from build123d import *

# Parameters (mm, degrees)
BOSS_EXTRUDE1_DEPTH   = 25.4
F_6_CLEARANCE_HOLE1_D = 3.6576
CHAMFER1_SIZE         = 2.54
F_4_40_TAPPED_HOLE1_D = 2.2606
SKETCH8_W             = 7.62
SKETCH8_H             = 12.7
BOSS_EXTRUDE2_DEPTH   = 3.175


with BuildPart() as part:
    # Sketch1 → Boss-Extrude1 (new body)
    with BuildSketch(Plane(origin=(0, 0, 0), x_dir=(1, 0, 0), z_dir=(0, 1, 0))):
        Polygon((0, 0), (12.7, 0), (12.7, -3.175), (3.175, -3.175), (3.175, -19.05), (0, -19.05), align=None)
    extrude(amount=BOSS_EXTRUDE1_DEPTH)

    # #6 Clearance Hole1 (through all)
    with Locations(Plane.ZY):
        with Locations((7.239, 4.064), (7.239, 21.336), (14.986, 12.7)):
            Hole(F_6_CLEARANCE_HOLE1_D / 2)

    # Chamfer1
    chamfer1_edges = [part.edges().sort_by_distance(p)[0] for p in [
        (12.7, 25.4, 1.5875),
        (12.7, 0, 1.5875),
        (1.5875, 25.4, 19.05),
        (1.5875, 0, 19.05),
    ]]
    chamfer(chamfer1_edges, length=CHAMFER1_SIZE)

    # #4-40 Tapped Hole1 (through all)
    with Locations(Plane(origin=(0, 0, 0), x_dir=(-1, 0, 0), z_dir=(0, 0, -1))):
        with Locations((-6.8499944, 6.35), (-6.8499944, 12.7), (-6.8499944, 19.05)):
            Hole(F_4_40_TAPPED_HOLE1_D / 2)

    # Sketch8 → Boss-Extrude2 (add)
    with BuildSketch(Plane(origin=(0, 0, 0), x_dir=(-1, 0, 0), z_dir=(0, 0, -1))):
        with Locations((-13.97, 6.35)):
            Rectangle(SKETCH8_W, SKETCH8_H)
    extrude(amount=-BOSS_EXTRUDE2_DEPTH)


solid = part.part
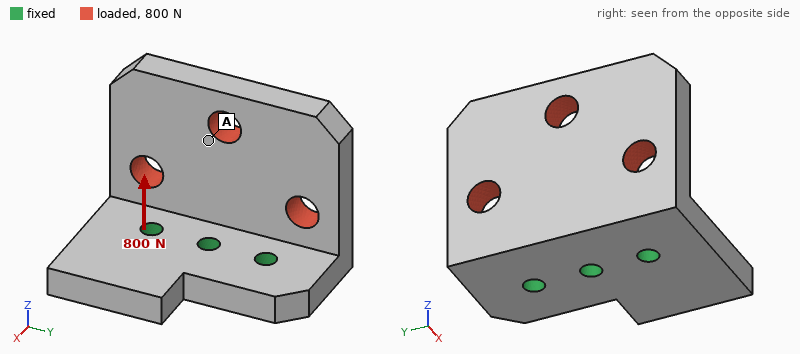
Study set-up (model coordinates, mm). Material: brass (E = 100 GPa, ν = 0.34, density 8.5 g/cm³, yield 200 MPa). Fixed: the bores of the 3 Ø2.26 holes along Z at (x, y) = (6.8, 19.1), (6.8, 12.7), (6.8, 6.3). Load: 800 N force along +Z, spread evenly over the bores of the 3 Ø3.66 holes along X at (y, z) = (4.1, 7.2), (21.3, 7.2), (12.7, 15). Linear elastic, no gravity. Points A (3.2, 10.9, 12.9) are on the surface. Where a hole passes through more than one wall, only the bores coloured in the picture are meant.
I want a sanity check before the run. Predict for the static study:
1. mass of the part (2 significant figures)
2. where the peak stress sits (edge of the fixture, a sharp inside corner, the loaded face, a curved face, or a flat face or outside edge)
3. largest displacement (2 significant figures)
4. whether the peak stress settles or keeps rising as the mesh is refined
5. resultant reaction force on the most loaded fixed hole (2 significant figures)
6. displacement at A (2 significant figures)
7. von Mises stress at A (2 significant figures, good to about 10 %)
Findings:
20 g
edge of the fixture
31 µm
keeps rising
280 N
20 µm
15 MPa
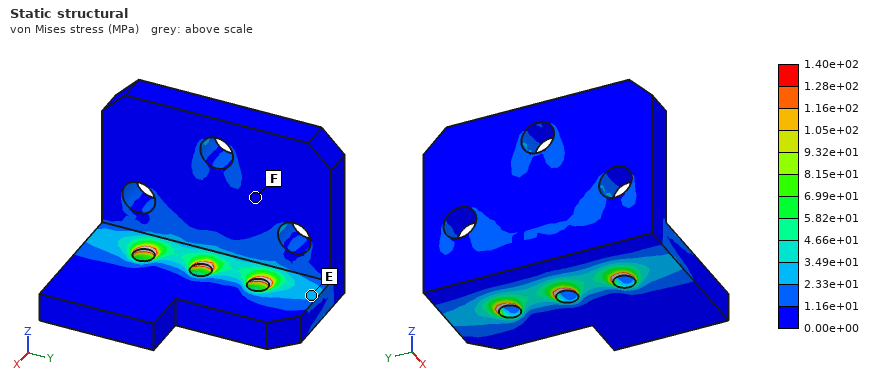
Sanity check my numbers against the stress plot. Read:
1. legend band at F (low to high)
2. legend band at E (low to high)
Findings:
0.00e+00 to 1.16e+01 MPa
2.33e+01 to 3.49e+01 MPa
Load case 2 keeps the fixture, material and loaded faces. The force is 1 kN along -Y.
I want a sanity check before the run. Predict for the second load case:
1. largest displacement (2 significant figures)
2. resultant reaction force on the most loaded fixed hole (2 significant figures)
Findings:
31 µm
710 N
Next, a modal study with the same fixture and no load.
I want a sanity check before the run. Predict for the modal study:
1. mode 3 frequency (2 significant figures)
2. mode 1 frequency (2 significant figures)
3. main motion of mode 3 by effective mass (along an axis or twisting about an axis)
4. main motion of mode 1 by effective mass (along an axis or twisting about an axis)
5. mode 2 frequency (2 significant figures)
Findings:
11 kHz
4200 Hz
along Y
along X
7900 Hz
